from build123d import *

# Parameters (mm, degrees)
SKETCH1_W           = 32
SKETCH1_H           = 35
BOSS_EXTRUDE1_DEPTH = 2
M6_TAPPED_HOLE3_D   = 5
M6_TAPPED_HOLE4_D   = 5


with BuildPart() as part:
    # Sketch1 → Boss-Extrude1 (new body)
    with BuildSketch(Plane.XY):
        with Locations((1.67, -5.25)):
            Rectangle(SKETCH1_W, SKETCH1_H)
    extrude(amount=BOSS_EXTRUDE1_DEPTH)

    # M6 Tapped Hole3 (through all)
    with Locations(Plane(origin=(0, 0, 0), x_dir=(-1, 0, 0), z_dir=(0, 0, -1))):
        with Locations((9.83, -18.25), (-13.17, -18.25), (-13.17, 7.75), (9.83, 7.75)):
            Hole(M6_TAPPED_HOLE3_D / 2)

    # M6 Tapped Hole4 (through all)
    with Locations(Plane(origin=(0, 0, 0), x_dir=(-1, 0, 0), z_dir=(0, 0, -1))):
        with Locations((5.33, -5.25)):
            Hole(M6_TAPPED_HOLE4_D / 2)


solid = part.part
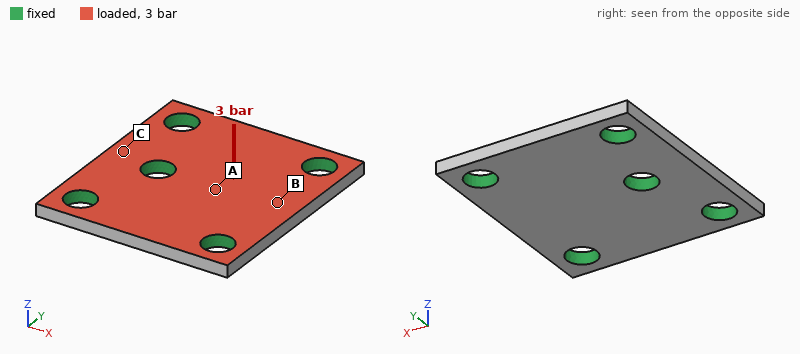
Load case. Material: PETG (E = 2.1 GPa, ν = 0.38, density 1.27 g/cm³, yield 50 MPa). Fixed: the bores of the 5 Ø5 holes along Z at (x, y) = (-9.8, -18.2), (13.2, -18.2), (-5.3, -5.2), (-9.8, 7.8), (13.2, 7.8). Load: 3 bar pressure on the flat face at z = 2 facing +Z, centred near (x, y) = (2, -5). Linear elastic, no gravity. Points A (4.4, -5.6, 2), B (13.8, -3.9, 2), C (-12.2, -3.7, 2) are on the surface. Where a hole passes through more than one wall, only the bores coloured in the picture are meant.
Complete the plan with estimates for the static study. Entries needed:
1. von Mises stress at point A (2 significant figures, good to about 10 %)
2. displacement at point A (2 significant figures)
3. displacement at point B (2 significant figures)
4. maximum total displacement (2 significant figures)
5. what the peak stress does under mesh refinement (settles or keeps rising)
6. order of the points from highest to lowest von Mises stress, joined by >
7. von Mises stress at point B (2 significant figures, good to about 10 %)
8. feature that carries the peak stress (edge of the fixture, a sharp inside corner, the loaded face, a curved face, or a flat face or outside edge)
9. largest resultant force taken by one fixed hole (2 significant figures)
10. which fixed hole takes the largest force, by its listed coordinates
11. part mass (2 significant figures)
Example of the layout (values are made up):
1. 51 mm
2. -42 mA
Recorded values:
1. 4.5 MPa
2. 0.10 mm
3. 0.13 mm
4. 0.15 mm
5. keeps rising
6. B > A > C
7. 7.7 MPa
8. edge of the fixture
9. 80 N
10. (-5.3, -5.2)
11. 2.6 g
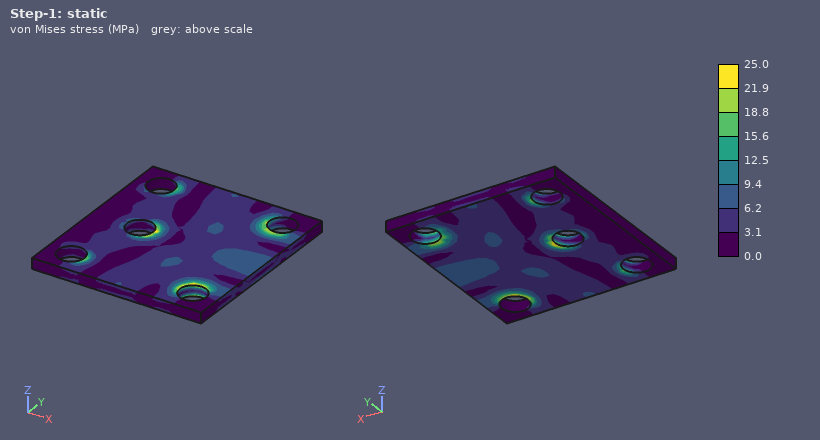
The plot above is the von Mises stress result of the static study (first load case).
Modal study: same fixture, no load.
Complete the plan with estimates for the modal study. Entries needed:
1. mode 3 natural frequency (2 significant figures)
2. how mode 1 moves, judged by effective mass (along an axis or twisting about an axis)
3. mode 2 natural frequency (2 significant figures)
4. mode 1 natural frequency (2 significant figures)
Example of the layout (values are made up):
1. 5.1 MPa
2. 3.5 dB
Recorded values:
1. 7200 Hz
2. along Z
3. 7000 Hz
4. 5400 Hz
